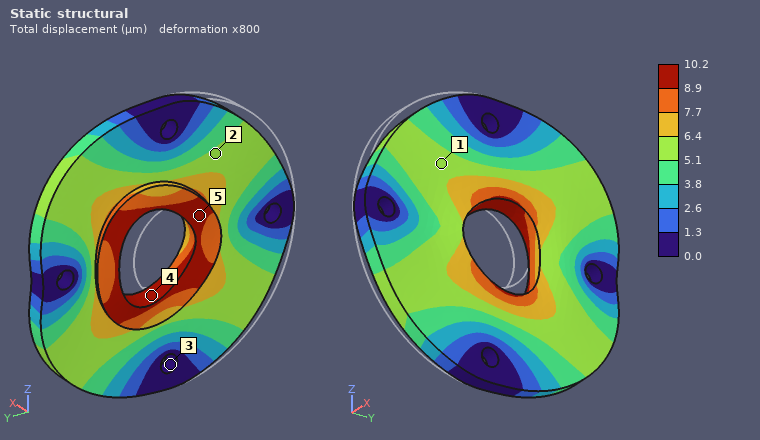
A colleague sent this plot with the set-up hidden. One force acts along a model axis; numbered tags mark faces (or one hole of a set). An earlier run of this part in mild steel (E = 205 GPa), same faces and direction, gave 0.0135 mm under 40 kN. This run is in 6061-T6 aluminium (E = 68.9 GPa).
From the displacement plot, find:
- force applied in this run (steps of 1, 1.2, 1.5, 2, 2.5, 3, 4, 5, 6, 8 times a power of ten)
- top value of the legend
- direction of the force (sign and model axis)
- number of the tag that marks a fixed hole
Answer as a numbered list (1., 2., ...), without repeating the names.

1. 10 kN
2. 10.2 µm
3. +Y
4. 3
